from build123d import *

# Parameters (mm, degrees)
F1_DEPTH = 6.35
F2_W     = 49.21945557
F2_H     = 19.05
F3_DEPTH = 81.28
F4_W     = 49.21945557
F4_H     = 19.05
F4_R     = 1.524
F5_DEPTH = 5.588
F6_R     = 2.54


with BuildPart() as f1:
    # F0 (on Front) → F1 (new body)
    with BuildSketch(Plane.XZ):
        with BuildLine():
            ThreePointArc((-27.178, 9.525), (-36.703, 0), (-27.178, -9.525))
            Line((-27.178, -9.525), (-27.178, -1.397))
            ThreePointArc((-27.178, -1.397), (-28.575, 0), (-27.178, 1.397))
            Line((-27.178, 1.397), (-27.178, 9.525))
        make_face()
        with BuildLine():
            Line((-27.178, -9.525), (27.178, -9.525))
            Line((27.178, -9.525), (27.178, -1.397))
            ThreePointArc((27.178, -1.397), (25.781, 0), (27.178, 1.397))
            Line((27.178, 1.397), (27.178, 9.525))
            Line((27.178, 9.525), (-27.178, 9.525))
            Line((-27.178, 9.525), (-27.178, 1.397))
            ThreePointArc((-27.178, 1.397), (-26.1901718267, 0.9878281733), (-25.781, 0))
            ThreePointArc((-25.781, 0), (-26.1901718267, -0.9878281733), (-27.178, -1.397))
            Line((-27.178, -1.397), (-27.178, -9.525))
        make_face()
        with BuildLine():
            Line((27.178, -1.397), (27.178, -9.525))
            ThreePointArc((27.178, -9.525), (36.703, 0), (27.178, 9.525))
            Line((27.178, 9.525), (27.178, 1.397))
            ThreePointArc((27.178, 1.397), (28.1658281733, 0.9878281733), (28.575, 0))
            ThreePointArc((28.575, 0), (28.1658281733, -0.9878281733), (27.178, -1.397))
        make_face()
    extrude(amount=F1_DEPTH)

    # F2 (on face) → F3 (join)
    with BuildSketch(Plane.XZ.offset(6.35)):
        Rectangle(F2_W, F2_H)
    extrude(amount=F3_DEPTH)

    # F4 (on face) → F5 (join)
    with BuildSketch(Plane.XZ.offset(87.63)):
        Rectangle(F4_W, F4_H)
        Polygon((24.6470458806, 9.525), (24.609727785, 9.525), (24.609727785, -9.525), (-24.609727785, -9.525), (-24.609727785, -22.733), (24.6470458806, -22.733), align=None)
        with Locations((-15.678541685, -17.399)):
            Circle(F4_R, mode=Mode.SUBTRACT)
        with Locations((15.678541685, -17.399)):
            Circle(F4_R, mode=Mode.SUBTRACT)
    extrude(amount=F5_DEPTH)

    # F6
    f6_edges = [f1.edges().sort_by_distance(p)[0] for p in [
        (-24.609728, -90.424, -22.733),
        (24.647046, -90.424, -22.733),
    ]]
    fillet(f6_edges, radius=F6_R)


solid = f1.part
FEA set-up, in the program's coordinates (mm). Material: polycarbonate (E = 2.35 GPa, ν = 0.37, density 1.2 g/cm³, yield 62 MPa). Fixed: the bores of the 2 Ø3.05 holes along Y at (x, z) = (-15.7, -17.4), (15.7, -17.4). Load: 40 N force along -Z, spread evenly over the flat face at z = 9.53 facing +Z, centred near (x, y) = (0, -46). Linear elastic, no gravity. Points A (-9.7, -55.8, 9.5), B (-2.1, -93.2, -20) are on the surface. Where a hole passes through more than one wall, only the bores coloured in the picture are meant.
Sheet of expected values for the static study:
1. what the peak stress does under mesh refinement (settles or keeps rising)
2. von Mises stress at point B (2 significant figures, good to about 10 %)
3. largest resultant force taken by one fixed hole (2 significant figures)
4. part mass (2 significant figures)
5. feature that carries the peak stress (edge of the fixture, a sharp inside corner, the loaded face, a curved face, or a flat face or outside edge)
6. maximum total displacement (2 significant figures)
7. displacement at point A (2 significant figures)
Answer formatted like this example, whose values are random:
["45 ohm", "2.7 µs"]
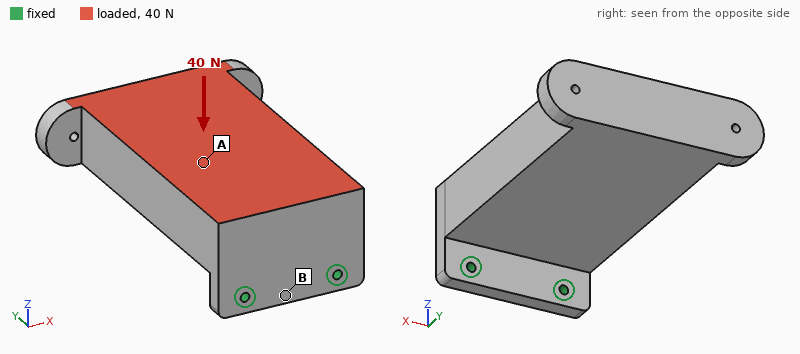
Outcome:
["keeps rising", "2.0 MPa", "21 N", "110 g", "edge of the fixture", "1.4 mm", "0.60 mm"]
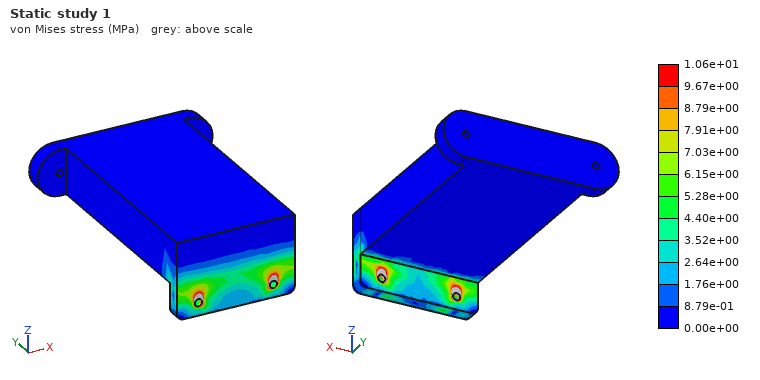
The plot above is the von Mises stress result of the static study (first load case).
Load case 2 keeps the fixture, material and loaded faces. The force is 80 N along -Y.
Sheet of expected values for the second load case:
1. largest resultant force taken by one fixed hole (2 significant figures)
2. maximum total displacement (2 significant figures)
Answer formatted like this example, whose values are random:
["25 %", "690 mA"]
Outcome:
["40 N", "1.4 mm"]
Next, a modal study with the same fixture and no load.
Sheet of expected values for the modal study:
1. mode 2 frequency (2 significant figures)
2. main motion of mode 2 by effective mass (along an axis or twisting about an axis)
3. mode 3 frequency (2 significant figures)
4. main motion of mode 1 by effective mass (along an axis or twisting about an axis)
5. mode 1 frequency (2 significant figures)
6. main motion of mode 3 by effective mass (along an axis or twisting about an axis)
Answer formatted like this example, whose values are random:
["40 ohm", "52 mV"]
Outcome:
["310 Hz", "along X", "1000 Hz", "along Z", "98 Hz", "along Y"]
